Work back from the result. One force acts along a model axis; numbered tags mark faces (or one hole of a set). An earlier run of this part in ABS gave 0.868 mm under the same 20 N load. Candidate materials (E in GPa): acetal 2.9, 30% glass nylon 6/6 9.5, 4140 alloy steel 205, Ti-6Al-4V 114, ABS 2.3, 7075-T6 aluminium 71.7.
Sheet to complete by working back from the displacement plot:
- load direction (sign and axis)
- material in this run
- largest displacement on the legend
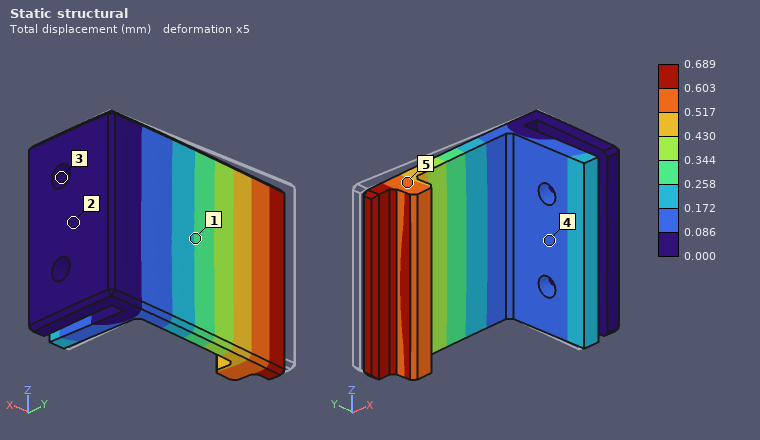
-Y
acetal
0.689 mm
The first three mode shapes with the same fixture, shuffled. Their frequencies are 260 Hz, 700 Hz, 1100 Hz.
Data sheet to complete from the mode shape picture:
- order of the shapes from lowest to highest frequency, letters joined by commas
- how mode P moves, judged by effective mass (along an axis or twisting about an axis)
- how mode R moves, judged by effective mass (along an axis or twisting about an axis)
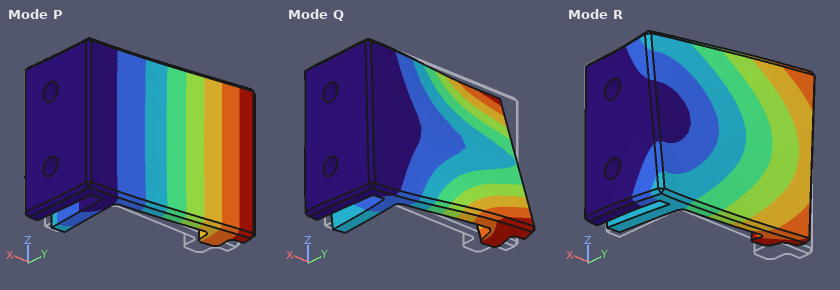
P, R, Q
along Y
along Z
